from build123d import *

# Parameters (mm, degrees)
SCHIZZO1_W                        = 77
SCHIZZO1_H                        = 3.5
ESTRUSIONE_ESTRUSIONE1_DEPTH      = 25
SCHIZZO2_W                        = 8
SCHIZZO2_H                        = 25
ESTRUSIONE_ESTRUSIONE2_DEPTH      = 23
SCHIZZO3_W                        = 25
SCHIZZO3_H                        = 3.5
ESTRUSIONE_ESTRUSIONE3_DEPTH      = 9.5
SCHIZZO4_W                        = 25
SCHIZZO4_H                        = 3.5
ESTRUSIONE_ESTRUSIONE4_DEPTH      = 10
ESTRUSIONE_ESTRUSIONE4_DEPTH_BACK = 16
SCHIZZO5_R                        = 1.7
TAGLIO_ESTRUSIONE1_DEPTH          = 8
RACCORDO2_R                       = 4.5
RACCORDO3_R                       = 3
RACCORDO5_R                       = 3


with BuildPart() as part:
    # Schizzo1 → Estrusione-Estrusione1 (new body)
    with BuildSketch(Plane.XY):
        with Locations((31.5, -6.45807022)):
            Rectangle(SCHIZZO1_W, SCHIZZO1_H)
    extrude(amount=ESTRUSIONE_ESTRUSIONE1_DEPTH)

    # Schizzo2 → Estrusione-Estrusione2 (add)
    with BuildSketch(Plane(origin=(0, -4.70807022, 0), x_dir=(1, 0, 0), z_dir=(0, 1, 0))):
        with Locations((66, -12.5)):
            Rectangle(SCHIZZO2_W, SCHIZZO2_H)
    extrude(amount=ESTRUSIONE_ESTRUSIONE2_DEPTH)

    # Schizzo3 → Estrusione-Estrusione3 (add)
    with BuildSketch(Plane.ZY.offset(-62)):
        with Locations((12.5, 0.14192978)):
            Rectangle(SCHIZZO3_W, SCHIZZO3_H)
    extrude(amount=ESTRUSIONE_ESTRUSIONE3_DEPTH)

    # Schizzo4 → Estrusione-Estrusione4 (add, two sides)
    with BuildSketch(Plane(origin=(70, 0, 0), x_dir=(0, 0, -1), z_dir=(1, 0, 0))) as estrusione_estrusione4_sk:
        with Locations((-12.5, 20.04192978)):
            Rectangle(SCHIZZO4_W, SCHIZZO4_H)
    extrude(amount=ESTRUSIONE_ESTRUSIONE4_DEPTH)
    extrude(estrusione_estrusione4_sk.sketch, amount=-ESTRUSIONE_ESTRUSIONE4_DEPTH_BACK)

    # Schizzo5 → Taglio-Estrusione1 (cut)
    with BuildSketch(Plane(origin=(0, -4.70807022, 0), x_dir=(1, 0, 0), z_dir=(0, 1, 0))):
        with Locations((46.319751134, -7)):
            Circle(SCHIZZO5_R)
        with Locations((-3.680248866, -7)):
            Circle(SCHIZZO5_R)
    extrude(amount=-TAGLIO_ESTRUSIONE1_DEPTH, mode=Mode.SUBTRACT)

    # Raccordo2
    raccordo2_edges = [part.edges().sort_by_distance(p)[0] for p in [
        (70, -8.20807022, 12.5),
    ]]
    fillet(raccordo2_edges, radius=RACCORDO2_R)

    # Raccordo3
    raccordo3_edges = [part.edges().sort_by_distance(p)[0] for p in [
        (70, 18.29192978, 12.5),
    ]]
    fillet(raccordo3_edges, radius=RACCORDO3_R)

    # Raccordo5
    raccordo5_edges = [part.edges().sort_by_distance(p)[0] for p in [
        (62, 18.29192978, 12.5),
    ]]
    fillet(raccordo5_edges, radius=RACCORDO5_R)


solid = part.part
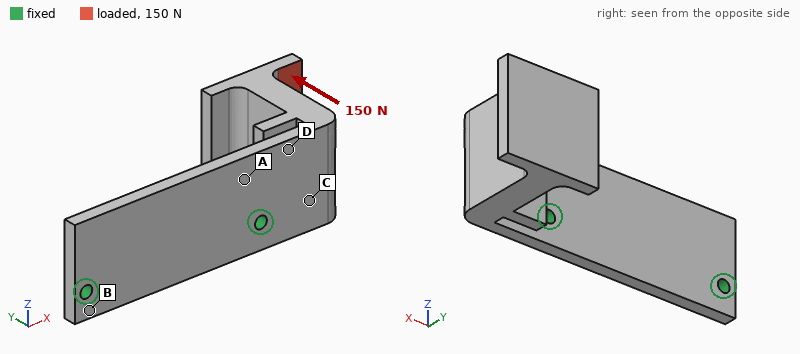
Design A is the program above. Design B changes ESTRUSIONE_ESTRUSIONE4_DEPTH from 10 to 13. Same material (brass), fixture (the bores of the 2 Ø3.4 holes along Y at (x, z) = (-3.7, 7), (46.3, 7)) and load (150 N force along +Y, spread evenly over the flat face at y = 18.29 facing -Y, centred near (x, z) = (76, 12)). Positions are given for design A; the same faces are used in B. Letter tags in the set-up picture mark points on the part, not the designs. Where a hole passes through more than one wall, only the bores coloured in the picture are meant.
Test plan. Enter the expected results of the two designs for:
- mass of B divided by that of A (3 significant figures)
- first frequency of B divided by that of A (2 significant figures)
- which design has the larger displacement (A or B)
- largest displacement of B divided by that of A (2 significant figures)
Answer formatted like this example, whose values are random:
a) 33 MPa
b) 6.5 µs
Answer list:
a) 1.02
b) 0.96
c) B
d) 1.1
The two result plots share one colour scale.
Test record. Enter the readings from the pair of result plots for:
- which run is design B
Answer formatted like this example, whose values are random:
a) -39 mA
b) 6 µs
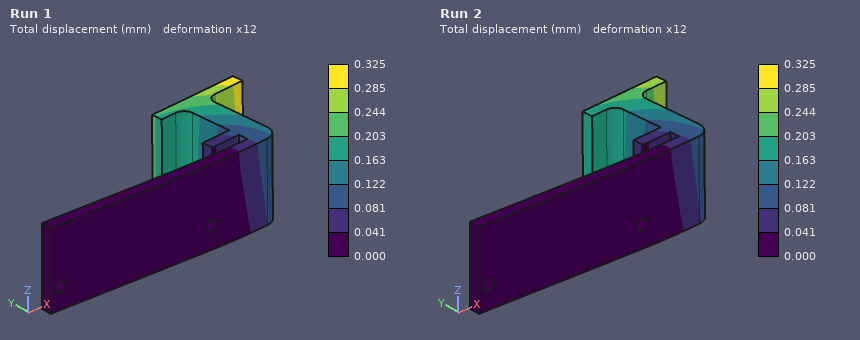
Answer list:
a) Run 1
